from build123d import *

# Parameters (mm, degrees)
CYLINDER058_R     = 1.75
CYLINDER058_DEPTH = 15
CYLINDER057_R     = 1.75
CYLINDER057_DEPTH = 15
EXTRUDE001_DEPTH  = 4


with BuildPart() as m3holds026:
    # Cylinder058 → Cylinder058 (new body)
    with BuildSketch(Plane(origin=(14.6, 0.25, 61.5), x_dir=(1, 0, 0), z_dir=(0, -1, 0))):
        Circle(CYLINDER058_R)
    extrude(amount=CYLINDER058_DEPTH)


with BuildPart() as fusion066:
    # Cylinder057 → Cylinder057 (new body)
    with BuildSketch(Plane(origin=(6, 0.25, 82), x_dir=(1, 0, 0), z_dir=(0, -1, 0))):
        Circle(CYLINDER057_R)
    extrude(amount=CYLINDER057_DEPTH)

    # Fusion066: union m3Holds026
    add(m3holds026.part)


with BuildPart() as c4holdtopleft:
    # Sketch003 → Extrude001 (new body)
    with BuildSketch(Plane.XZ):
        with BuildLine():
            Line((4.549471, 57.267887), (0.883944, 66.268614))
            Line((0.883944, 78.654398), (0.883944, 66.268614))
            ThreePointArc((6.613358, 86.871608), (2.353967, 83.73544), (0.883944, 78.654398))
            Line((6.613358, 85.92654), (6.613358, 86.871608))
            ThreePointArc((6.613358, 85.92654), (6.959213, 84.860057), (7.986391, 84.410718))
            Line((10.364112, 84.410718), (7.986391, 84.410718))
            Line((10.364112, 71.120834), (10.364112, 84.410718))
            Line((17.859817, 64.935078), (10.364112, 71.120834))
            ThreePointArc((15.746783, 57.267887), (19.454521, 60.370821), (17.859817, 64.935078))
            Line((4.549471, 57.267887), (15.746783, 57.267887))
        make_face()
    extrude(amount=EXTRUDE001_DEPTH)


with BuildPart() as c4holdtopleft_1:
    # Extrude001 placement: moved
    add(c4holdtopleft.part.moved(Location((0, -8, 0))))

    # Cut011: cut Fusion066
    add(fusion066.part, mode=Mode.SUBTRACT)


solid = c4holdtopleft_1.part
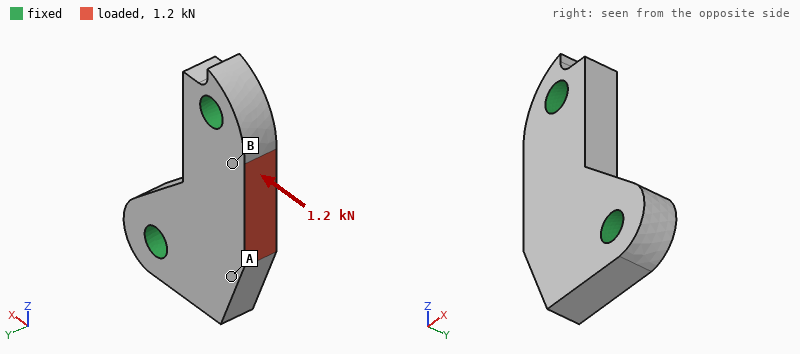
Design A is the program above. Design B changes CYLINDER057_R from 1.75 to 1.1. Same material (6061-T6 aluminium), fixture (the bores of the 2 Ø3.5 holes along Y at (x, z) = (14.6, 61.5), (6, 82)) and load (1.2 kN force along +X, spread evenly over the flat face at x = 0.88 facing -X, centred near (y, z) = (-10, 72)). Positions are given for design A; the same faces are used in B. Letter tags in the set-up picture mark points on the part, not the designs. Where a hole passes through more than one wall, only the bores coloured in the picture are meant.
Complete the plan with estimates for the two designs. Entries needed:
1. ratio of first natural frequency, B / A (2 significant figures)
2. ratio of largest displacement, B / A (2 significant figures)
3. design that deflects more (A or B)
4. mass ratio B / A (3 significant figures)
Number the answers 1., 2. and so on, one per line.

1. 0.95
2. 1.1
3. B
4. 1.02
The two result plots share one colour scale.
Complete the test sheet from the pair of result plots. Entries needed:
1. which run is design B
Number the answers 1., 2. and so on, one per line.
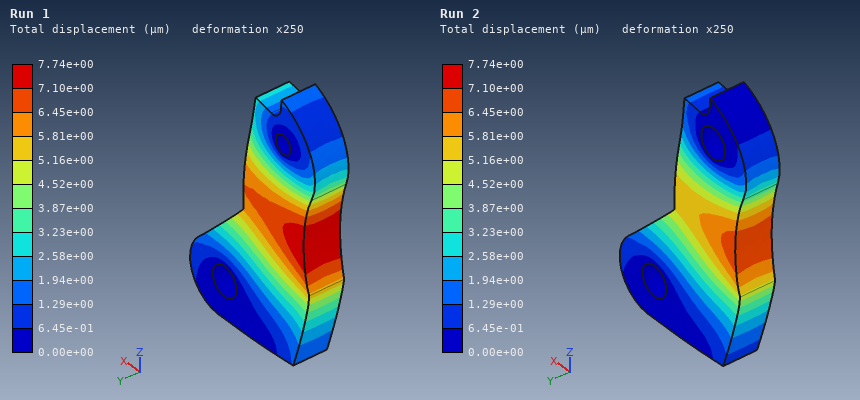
1. Run 1
